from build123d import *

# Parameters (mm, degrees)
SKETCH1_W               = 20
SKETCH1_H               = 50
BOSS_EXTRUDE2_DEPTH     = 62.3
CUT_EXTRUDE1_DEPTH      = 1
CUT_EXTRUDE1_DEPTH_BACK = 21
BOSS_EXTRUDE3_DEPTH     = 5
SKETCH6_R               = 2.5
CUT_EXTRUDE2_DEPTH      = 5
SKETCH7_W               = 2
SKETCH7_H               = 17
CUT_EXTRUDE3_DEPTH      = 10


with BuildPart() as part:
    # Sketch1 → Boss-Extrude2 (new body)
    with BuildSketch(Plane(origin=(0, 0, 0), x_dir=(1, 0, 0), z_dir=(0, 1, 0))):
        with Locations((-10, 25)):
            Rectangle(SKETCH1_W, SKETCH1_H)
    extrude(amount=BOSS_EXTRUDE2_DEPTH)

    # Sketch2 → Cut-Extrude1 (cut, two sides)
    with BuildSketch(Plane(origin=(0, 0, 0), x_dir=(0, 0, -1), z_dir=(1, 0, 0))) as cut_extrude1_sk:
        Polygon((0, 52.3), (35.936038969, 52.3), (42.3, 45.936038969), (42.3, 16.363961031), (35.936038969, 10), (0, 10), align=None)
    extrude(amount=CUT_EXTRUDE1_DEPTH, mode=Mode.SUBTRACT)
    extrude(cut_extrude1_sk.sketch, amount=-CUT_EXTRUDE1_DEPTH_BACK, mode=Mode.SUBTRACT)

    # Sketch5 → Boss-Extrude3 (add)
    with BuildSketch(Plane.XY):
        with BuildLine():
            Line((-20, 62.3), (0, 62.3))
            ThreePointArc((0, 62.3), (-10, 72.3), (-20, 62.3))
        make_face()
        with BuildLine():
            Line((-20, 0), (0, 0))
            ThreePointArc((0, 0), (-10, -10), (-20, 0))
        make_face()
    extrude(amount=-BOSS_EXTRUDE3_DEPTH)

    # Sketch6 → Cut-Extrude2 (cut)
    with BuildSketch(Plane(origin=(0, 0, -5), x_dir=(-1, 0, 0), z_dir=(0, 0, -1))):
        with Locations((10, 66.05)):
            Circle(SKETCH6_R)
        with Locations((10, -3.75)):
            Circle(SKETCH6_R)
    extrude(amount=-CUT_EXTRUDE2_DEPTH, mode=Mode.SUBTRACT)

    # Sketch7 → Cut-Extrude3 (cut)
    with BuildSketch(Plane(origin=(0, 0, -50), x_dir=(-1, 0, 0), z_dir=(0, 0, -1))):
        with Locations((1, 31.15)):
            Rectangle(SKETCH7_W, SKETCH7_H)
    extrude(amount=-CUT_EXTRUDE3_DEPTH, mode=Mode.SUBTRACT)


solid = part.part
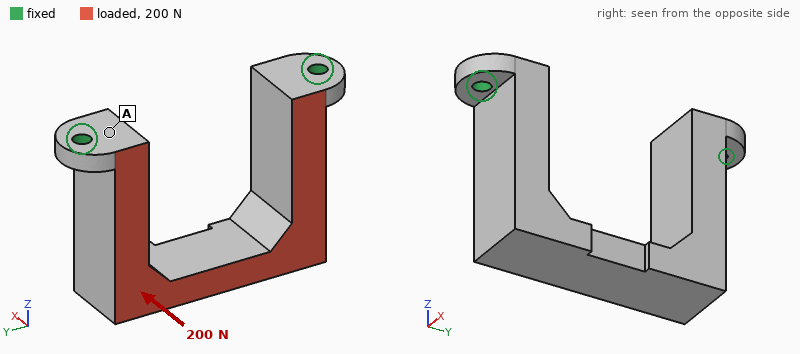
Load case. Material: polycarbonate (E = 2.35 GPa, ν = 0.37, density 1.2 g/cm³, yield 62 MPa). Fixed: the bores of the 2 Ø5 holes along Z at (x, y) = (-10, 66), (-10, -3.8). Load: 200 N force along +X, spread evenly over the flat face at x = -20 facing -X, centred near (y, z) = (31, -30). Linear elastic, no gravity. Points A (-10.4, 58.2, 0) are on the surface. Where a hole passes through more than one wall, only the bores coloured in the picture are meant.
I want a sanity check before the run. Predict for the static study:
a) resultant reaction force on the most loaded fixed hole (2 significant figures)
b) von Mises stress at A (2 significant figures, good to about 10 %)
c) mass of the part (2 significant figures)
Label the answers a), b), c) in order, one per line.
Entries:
a) 100 N
b) 6.2 MPa
c) 34 g
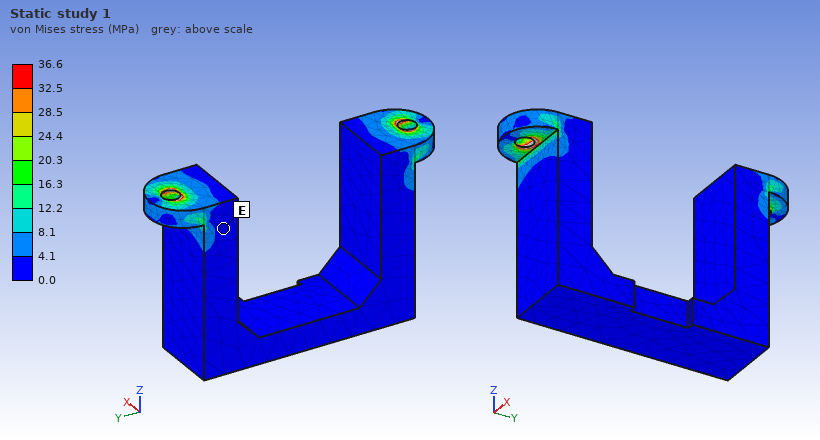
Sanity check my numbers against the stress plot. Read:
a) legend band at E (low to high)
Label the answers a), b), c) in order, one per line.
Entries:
a) 0.0 to 4.1 MPa
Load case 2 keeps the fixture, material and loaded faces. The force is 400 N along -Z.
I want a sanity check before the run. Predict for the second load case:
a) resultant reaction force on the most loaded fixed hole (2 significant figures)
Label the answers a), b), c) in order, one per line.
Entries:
a) 200 N
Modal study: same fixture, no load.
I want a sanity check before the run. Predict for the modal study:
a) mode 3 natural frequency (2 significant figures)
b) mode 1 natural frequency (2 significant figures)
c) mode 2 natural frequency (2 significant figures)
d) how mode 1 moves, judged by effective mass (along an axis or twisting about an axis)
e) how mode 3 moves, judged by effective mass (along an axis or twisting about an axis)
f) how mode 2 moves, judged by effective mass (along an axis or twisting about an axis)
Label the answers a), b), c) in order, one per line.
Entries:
a) 1000 Hz
b) 450 Hz
c) 780 Hz
d) along X
e) twisting about Z
f) along Y
